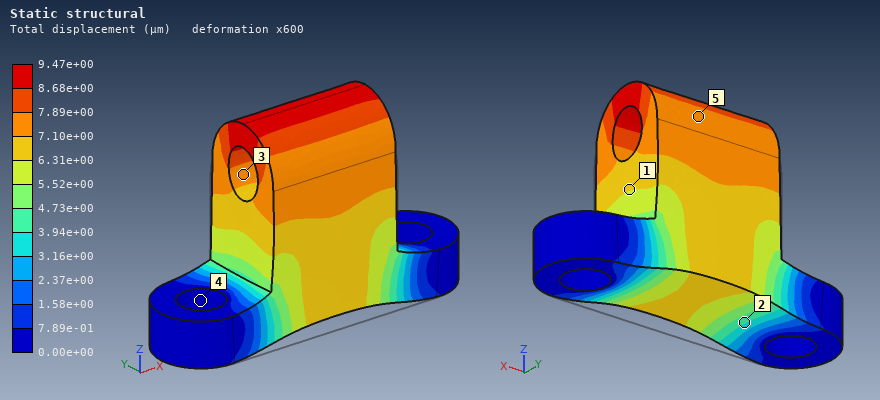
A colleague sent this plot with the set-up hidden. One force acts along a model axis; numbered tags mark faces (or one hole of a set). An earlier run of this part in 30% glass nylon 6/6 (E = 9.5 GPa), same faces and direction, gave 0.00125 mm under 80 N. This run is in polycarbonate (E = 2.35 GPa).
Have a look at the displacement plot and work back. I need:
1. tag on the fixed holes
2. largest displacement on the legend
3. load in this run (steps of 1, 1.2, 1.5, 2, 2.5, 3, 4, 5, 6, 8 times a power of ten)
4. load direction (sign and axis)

4
9.47e+00 µm
150 N
+Z
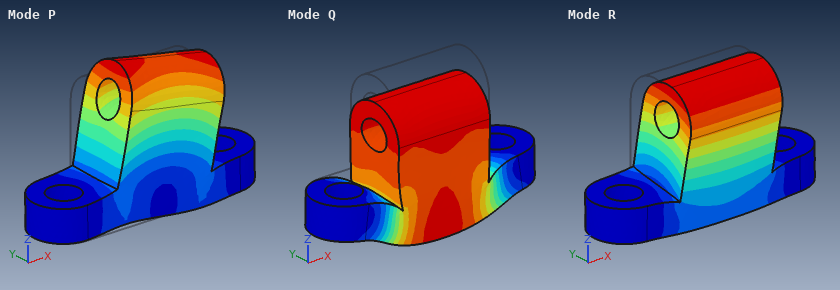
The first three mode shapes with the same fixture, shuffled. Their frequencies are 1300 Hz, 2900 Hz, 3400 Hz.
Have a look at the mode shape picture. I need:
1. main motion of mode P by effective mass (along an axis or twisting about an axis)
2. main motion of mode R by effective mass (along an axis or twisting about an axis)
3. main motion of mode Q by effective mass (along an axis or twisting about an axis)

along X
along Y
along Z
